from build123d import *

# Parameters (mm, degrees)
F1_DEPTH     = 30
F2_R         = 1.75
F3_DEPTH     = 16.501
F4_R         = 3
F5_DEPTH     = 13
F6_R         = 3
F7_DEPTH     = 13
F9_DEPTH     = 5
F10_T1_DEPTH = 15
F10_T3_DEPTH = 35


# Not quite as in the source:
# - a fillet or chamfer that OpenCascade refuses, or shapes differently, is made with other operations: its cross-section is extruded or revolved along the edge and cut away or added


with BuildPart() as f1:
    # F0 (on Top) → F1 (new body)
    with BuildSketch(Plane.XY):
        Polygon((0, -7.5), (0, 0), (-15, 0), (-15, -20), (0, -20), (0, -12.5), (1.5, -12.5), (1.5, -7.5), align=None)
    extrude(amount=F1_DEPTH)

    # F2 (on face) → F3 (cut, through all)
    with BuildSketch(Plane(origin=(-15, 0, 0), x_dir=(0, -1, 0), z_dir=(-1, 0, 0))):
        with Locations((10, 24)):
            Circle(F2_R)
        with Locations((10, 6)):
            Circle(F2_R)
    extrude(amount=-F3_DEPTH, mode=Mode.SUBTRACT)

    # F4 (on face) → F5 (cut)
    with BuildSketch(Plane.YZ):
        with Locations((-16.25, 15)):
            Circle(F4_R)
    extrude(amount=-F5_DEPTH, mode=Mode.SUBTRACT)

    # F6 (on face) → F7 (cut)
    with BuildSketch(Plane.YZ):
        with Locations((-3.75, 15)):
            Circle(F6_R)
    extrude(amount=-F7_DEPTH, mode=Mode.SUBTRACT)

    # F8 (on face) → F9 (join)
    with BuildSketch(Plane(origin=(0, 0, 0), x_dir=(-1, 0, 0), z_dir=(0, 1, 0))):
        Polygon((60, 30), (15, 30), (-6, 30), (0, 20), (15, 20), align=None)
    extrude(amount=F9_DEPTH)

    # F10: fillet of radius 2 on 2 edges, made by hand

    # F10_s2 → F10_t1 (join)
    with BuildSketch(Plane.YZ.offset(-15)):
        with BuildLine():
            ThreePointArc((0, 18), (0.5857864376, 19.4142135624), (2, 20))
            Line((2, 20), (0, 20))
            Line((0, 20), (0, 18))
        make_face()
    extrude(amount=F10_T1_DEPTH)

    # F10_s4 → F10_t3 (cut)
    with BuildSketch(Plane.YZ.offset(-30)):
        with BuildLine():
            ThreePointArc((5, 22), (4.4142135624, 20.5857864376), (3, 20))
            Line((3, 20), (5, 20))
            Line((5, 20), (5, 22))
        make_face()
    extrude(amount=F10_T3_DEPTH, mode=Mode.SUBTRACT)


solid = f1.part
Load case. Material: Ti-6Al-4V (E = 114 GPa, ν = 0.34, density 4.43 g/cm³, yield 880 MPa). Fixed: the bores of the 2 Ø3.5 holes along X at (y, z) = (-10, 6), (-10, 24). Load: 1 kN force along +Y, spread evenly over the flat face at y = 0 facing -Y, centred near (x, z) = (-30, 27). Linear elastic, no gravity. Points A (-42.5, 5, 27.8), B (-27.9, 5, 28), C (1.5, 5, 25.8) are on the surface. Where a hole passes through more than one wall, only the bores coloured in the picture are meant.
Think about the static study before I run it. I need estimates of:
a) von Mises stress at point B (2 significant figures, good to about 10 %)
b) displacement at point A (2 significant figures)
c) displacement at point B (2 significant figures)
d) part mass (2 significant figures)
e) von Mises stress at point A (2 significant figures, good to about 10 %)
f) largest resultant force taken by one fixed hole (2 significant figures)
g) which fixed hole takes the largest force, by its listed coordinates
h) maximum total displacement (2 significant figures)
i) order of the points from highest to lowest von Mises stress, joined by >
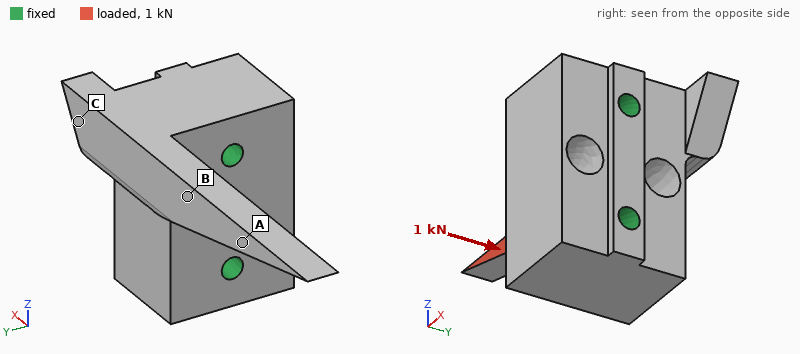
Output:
190 MPa
0.47 mm
0.17 mm
45 g
56 MPa
1.1 kN
(-10, 24)
0.88 mm
B > A > C
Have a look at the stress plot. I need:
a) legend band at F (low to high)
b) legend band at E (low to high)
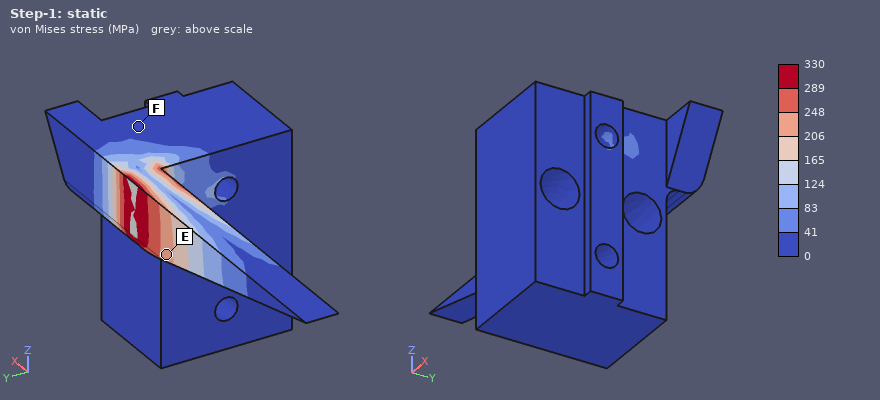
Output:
0 to 41 MPa
206 to 248 MPa
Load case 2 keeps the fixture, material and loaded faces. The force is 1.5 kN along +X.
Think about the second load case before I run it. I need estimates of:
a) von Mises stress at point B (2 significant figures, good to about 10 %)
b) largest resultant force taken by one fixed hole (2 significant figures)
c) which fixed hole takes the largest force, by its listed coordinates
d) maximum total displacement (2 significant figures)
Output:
34 MPa
1.5 kN
(-10, 24)
0.25 mm
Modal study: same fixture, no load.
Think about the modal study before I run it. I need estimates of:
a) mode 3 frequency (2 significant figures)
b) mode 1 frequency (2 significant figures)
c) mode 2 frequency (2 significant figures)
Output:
14 kHz
3500 Hz
5000 Hz
